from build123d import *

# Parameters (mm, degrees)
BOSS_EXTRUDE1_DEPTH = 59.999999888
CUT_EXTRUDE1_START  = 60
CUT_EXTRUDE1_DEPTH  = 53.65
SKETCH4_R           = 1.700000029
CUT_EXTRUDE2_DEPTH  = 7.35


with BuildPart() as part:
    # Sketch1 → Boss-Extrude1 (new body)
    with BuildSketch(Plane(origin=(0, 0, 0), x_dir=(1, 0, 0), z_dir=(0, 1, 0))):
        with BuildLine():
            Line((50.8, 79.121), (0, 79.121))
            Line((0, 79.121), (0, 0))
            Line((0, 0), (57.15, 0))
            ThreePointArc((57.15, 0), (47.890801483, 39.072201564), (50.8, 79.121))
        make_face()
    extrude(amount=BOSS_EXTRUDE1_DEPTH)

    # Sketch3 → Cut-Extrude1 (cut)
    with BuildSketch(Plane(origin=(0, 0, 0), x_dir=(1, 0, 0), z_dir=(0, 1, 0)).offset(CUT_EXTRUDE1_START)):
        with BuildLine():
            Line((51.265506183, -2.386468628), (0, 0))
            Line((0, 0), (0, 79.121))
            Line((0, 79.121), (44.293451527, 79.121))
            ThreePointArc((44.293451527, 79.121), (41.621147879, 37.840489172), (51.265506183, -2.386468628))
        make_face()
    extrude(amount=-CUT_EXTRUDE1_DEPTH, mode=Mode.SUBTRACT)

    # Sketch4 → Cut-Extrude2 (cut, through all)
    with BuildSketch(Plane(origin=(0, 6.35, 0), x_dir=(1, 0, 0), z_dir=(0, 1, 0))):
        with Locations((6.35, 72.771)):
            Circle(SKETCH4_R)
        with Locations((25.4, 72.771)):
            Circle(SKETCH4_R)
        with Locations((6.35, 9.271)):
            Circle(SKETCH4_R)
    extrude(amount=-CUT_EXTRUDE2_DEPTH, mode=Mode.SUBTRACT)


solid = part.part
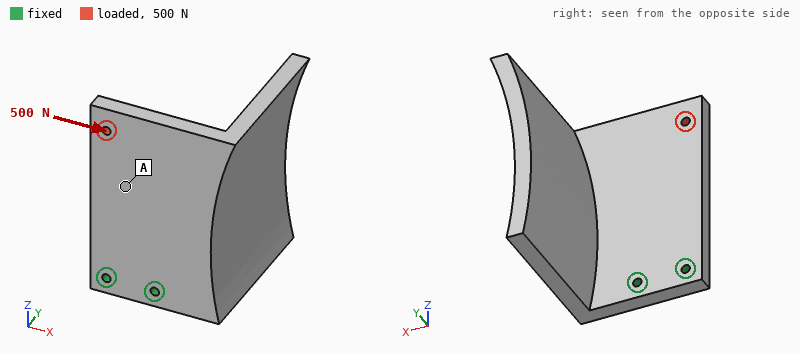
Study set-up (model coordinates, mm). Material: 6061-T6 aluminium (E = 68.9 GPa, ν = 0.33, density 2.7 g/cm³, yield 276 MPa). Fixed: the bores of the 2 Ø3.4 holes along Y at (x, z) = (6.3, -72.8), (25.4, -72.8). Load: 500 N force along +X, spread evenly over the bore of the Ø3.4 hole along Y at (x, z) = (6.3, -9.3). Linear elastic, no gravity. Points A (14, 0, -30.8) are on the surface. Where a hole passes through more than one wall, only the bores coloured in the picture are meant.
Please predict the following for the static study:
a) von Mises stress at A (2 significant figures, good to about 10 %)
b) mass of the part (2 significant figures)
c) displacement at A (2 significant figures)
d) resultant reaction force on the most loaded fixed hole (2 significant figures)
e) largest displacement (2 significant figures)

3.9 MPa
140 g
21 µm
1.5 kN
44 µm
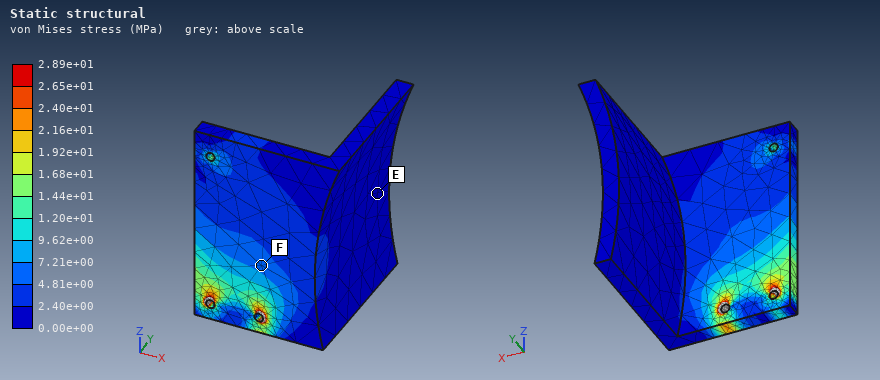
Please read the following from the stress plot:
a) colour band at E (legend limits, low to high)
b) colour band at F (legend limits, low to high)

0.00e+00 to 2.40e+00 MPa
4.81e+00 to 7.21e+00 MPa
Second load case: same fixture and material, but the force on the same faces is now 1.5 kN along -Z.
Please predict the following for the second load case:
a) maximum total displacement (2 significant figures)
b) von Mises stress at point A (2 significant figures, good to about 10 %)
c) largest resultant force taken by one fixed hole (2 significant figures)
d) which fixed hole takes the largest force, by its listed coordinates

29 µm
8.5 MPa
1.4 kN
(6.3, -72.8)
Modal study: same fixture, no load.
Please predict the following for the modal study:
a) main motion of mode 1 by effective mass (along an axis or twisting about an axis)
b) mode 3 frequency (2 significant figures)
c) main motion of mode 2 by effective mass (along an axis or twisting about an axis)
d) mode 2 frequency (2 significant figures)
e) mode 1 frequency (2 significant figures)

along Y
2200 Hz
along X
860 Hz
520 Hz
